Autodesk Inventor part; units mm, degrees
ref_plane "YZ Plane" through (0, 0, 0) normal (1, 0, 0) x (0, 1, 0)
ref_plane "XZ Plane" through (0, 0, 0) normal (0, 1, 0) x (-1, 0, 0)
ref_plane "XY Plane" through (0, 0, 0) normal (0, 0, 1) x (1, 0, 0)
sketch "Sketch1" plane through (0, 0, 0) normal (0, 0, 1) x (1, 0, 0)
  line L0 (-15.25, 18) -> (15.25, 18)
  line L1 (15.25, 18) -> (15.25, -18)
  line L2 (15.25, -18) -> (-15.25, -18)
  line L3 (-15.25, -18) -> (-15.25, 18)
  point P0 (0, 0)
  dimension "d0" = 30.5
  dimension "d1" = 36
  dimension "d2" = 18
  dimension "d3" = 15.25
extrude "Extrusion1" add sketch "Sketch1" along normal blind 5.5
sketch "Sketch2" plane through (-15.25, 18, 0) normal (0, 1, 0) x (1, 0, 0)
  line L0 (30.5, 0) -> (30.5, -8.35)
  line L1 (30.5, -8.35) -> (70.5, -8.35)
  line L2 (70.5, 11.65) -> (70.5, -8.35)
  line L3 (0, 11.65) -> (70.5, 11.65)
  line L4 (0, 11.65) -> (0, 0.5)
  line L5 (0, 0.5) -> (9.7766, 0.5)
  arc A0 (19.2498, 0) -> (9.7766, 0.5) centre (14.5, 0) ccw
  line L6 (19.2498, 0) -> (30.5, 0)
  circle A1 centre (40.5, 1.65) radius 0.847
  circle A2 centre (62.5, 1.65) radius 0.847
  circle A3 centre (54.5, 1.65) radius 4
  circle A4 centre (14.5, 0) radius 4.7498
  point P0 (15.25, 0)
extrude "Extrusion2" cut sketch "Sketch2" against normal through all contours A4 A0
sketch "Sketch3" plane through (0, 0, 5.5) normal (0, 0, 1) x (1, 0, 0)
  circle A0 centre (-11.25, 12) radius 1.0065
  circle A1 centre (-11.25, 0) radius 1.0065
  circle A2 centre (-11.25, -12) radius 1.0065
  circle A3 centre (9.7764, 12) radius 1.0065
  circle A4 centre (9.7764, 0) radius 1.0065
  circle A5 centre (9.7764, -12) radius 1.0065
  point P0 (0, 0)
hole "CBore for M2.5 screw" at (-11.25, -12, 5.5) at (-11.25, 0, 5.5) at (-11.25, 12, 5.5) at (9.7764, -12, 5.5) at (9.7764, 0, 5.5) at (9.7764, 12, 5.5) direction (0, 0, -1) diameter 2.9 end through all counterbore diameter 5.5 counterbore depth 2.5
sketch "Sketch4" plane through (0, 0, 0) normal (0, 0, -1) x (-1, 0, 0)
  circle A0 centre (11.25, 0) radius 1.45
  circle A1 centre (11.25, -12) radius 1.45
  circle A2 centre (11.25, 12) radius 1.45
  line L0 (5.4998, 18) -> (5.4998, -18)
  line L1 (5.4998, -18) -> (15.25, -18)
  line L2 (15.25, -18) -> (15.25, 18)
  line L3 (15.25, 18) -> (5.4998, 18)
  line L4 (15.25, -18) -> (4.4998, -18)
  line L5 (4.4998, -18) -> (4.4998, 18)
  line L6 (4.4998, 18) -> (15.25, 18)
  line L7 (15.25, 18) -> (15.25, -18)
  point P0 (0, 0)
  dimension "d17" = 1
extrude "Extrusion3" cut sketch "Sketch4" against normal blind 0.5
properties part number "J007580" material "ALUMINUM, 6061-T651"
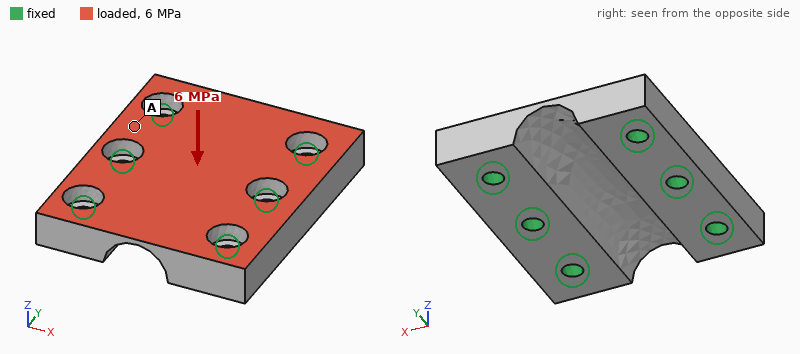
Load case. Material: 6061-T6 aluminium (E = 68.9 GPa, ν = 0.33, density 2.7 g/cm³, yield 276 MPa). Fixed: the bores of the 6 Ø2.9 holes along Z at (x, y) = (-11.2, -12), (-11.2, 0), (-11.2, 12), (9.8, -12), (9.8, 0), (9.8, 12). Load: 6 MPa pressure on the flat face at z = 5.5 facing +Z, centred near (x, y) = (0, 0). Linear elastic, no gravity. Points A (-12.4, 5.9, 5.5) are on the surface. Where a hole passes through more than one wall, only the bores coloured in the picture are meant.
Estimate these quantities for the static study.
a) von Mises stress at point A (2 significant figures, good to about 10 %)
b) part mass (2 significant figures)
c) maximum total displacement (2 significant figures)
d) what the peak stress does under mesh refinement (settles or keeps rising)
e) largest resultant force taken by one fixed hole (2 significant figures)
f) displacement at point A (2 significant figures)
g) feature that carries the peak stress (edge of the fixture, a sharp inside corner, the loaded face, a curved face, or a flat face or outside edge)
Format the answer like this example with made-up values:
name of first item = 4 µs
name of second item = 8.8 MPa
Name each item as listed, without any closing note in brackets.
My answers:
von Mises stress at point A = 14 MPa
part mass = 11 g
maximum total displacement = 19 µm
what the peak stress does under mesh refinement = keeps rising
largest resultant force taken by one fixed hole = 1.2 kN
displacement at point A = 3.1 µm
feature that carries the peak stress = edge of the fixture
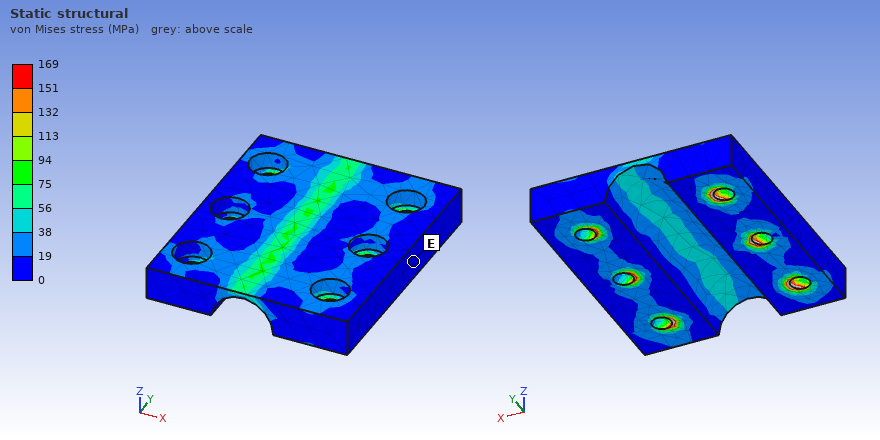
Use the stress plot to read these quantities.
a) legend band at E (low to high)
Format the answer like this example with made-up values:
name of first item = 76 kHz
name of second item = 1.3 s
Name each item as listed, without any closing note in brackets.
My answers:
legend band at E = 0 to 19 MPa
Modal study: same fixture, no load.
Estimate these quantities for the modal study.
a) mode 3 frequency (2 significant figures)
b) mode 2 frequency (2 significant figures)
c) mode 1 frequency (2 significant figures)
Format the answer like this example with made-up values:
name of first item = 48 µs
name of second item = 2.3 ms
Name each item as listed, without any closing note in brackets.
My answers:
mode 3 frequency = 44 kHz
mode 2 frequency = 43 kHz
mode 1 frequency = 42 kHz
